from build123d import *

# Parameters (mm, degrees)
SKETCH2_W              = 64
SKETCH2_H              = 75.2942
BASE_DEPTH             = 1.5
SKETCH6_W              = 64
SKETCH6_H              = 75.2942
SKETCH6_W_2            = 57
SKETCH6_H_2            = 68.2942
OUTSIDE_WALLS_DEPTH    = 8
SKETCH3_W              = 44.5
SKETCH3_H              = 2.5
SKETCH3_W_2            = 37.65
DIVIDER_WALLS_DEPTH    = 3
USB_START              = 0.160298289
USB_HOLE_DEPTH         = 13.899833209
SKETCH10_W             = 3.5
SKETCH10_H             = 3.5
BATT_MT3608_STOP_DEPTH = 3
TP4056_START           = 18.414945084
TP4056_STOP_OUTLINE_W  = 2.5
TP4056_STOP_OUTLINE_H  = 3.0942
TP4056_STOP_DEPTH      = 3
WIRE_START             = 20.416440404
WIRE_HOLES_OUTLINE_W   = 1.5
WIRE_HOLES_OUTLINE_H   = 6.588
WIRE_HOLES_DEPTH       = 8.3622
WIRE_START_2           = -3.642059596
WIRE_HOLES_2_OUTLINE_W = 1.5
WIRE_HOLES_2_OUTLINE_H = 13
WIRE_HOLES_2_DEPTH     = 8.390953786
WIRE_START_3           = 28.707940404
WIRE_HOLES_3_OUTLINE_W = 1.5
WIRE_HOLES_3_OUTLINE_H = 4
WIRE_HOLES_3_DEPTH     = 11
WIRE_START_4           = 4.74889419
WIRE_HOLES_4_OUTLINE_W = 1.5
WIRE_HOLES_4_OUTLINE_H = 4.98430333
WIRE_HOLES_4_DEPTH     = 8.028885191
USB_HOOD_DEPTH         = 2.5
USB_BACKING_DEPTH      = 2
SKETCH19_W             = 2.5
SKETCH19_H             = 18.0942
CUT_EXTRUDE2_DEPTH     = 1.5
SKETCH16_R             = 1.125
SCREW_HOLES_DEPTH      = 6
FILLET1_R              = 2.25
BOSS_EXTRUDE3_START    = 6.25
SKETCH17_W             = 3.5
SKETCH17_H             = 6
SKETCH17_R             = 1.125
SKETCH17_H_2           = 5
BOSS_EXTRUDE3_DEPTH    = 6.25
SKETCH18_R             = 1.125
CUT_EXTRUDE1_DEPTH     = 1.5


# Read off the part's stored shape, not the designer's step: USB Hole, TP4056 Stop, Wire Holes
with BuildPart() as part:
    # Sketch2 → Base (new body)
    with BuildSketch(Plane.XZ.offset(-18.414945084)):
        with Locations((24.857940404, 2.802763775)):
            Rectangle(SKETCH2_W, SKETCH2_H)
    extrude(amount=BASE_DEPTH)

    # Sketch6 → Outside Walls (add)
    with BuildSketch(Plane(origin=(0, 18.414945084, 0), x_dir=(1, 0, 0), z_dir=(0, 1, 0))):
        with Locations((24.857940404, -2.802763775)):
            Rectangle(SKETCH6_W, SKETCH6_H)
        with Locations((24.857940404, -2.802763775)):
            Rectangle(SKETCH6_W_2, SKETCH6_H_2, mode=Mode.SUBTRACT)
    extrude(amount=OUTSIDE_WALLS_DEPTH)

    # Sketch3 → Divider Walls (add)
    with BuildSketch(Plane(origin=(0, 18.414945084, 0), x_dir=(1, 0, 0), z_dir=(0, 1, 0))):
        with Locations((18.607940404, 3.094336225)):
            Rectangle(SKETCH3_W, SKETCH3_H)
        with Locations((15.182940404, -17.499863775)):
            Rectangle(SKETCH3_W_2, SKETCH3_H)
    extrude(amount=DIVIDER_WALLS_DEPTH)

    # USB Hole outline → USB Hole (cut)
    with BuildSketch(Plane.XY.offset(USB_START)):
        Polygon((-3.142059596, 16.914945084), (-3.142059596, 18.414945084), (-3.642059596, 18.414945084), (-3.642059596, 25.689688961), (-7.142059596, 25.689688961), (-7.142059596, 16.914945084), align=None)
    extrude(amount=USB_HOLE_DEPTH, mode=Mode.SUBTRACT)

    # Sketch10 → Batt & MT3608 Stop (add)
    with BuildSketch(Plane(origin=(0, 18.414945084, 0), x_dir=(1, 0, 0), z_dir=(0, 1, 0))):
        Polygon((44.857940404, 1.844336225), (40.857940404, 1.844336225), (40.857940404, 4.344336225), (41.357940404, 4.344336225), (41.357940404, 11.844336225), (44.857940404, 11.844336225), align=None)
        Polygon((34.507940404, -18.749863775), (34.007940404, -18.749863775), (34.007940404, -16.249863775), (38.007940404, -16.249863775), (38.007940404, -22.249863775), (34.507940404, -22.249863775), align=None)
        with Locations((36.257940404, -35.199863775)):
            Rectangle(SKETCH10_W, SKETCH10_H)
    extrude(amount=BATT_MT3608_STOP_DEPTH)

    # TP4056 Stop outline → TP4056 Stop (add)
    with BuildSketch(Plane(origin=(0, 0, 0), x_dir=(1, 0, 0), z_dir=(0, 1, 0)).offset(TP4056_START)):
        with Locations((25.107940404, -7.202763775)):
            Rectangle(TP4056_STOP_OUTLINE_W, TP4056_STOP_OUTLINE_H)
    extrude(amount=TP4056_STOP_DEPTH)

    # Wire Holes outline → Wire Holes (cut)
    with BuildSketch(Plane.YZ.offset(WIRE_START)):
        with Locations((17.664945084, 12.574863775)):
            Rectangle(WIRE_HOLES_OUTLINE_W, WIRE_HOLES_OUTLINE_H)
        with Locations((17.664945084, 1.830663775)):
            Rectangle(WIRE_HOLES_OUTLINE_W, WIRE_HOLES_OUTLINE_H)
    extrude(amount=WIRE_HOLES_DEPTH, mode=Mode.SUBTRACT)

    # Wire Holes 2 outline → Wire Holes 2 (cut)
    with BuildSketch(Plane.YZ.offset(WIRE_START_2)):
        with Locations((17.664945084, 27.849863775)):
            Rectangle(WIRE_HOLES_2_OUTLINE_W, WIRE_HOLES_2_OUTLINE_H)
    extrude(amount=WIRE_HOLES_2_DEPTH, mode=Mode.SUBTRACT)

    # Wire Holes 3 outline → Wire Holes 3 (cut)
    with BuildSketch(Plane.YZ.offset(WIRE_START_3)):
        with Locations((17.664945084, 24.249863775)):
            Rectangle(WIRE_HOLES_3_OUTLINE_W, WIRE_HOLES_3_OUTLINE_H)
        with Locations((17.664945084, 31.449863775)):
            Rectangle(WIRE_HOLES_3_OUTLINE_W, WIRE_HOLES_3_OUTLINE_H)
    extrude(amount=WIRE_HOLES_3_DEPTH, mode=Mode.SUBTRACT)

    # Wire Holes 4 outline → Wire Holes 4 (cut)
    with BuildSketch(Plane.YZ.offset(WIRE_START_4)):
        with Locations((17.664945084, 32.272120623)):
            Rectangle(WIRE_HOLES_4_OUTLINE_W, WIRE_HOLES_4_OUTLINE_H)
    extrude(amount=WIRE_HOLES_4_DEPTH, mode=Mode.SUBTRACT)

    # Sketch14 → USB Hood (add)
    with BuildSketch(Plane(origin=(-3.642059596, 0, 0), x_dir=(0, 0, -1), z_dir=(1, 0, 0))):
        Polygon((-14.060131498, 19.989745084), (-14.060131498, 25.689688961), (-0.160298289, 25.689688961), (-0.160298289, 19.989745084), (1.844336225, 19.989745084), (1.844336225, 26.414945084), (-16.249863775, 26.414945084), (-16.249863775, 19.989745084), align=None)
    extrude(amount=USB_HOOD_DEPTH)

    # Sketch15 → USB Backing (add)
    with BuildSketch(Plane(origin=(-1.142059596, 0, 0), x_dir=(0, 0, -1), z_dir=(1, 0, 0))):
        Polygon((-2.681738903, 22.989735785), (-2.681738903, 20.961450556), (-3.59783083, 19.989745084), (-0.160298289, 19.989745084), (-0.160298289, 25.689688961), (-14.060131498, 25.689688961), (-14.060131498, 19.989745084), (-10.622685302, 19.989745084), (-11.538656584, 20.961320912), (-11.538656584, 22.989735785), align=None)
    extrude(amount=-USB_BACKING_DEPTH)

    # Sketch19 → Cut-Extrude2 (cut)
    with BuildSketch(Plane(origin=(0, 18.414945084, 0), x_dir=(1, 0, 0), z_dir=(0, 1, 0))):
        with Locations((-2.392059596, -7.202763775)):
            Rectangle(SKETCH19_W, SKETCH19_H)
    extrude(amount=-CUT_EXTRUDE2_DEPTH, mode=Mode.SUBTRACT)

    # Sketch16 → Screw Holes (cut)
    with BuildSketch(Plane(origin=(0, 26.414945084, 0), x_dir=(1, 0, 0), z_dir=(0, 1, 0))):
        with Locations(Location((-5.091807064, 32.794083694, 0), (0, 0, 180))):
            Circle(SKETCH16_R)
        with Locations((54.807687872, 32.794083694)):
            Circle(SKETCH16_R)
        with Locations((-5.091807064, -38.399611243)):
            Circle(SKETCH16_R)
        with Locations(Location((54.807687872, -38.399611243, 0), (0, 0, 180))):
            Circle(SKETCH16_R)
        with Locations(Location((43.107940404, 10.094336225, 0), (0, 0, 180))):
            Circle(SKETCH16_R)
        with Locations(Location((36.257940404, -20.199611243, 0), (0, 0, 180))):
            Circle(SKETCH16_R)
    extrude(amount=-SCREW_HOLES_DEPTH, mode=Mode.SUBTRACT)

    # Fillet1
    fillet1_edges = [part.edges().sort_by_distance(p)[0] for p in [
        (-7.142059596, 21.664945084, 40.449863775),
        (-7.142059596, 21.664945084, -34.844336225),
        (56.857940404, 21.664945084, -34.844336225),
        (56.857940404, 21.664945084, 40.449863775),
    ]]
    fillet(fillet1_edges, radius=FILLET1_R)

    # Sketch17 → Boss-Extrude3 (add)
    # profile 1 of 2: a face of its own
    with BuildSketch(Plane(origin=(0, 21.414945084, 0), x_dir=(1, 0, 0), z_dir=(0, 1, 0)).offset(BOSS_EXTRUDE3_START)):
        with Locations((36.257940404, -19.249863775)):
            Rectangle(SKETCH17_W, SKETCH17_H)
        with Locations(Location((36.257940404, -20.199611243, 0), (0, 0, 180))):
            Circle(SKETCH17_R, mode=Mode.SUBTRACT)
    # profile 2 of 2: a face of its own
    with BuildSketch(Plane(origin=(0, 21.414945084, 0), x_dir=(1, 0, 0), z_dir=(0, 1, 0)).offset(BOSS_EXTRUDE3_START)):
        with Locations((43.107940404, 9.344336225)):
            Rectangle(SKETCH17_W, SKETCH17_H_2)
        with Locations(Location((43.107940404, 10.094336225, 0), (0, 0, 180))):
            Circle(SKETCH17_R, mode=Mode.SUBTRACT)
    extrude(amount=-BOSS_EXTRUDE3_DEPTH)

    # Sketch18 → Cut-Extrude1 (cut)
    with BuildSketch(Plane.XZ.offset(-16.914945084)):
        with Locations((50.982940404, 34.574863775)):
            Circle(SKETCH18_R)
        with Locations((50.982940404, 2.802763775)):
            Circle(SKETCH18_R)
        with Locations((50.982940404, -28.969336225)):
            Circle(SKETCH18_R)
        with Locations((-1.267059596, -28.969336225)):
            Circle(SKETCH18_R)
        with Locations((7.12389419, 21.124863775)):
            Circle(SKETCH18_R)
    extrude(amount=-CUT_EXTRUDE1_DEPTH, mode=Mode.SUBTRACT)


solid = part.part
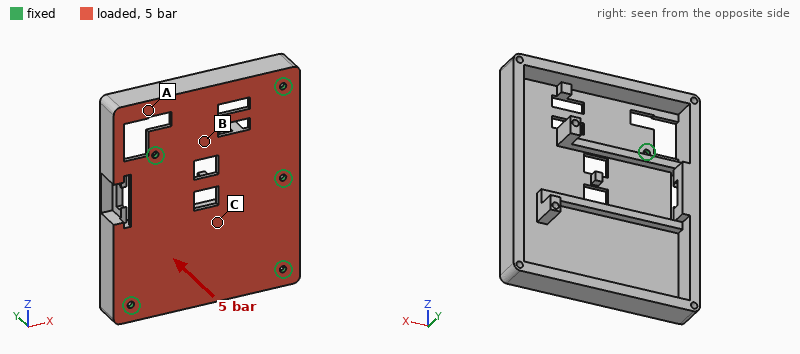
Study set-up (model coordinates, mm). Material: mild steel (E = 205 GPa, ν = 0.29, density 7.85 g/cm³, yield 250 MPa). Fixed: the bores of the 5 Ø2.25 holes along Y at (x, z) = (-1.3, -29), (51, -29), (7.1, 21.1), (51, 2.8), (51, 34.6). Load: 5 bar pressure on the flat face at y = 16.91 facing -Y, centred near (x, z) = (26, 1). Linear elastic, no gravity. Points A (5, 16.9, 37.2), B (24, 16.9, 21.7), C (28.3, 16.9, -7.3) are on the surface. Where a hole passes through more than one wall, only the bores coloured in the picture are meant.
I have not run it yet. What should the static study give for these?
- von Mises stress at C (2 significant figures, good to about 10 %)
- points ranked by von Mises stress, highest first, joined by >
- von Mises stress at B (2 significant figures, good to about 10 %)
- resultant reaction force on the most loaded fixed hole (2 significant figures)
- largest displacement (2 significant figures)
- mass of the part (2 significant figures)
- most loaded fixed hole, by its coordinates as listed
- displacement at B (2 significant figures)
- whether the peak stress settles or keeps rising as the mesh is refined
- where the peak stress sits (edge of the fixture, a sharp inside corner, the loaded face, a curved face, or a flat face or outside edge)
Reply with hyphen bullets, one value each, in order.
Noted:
- 53 MPa
- C > B > A
- 34 MPa
- 700 N
- 73 µm
- 120 g
- (7.1, 21.1)
- 29 µm
- keeps rising
- edge of the fixture
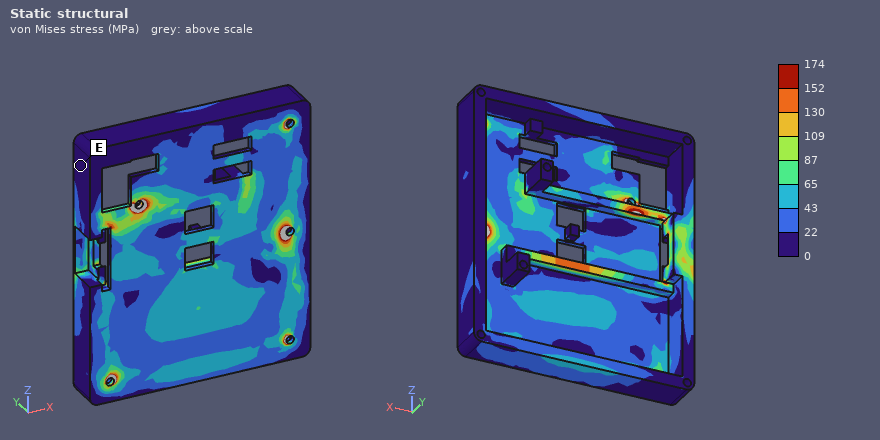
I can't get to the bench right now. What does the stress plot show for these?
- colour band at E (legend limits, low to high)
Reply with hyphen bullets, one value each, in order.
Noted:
- 0 to 22 MPa
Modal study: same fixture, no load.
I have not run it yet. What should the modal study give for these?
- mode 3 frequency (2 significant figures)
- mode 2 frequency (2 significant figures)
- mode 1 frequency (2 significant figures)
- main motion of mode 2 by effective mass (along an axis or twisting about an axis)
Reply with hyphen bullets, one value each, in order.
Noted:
- 5300 Hz
- 4100 Hz
- 2800 Hz
- along Y
